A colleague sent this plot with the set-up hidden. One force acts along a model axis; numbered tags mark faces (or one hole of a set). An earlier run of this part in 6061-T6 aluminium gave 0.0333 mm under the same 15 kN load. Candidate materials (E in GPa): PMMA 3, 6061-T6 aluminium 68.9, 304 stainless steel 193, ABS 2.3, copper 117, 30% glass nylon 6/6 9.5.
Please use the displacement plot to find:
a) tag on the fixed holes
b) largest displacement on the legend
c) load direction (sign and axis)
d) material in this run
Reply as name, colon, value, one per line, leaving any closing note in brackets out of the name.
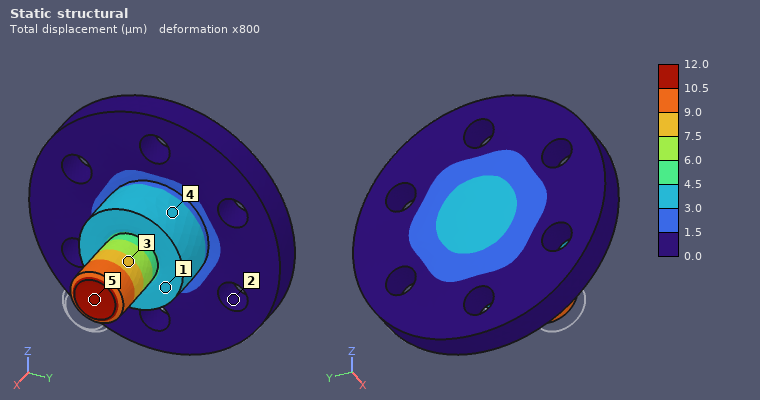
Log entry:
tag on the fixed holes: 2
largest displacement on the legend: 12.0 µm
load direction: -X
material in this run: 304 stainless steel
